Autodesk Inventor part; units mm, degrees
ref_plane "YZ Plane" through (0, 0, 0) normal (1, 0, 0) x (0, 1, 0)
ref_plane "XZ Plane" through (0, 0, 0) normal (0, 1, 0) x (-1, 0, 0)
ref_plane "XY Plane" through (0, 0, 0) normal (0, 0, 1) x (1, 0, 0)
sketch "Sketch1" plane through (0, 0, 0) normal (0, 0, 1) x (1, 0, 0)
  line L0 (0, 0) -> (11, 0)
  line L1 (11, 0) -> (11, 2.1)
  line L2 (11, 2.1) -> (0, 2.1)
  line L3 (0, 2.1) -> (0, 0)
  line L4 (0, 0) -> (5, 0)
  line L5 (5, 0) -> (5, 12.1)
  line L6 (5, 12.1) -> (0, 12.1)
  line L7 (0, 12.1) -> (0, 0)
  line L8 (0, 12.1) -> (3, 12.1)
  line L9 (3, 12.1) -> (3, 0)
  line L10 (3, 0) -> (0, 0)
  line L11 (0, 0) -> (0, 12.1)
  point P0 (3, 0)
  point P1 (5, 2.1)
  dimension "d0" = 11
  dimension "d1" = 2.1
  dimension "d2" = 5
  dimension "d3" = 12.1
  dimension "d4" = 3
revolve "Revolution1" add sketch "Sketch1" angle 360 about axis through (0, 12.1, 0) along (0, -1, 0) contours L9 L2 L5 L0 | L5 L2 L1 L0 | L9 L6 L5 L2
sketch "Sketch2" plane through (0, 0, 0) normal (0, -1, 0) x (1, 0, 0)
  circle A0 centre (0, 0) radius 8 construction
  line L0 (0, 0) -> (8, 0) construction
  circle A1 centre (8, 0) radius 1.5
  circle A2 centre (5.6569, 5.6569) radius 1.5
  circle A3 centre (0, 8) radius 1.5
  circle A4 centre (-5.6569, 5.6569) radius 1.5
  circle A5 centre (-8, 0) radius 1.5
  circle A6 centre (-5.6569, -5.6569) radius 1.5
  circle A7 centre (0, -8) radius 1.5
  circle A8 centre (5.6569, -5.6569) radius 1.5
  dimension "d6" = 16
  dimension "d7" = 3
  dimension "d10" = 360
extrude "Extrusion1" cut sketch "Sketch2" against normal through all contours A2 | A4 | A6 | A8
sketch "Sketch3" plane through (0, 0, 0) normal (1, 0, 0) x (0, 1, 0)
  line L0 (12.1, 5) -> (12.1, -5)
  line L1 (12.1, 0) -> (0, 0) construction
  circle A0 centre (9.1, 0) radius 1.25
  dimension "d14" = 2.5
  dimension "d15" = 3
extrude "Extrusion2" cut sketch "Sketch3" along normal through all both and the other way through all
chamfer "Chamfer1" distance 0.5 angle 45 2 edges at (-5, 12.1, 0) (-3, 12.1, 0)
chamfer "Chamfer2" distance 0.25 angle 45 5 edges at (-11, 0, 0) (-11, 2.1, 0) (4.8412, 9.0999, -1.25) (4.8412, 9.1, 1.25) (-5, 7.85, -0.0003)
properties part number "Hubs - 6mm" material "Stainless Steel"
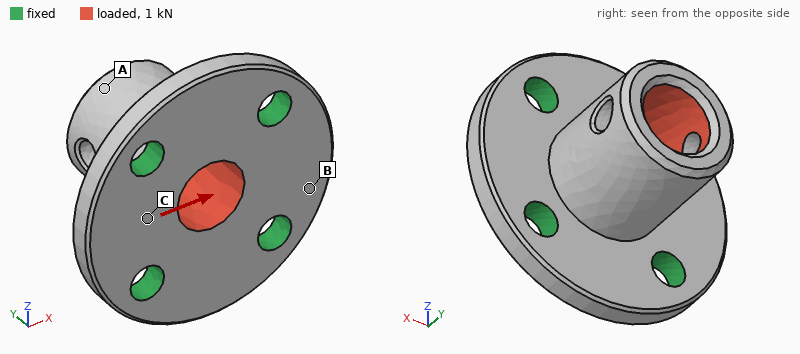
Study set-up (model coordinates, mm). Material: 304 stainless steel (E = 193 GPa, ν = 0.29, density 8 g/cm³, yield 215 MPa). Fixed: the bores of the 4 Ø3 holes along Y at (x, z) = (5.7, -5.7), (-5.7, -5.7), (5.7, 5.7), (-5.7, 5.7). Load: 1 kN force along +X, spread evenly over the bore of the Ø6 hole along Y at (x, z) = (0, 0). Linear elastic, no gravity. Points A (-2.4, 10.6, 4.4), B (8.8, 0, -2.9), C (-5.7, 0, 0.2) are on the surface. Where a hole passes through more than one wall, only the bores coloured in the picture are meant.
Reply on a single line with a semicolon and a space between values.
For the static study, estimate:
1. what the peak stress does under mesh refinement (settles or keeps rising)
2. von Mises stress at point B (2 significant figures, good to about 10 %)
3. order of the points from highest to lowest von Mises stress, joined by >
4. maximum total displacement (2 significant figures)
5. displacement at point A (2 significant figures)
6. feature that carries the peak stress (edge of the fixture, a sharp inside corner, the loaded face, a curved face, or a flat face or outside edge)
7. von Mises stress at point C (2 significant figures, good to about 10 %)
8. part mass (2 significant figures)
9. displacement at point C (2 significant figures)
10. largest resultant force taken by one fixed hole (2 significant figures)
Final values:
keeps rising; 16 MPa; C > B > A; 6.9 µm; 5.7 µm; edge of the fixture; 28 MPa; 9.2 g; 1.4 µm; 360 N
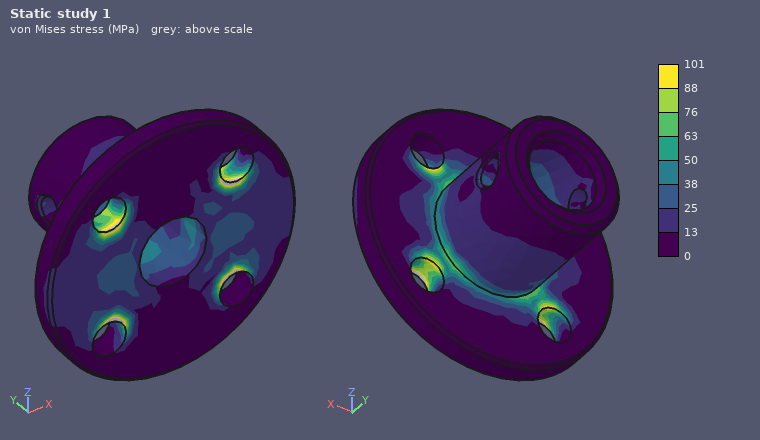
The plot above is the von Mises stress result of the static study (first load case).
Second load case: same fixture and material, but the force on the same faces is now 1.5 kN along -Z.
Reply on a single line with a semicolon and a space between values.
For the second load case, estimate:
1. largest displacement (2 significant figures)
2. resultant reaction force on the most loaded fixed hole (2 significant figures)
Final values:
11 µm; 530 N
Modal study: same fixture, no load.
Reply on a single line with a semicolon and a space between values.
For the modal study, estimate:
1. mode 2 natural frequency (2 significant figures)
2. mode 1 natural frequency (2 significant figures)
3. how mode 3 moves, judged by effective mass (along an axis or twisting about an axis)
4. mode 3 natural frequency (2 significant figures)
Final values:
32 kHz; 31 kHz; along Y; 54 kHz
